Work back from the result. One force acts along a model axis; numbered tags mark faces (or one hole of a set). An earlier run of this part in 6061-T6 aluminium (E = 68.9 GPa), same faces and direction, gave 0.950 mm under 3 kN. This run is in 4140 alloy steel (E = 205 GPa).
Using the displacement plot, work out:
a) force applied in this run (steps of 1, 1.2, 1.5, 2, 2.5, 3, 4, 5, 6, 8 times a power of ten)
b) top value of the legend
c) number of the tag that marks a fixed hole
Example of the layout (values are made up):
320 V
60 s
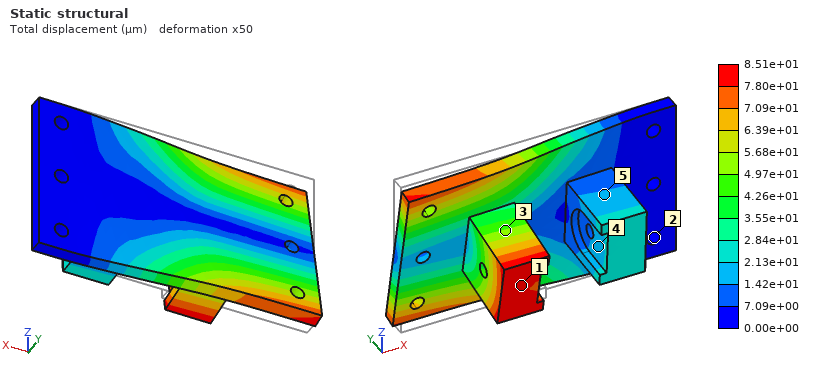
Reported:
800 N
8.51e+01 µm
2
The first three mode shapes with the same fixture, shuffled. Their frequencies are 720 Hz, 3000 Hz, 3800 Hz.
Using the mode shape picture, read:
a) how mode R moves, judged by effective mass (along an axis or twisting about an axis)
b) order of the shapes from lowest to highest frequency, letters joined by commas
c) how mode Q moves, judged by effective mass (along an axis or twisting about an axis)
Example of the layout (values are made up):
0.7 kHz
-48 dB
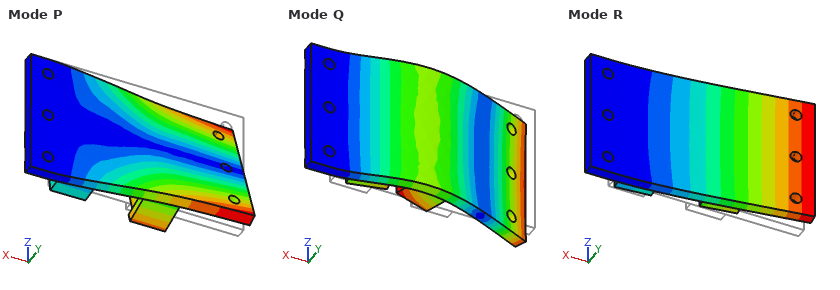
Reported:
along Y
R, P, Q
along Y
